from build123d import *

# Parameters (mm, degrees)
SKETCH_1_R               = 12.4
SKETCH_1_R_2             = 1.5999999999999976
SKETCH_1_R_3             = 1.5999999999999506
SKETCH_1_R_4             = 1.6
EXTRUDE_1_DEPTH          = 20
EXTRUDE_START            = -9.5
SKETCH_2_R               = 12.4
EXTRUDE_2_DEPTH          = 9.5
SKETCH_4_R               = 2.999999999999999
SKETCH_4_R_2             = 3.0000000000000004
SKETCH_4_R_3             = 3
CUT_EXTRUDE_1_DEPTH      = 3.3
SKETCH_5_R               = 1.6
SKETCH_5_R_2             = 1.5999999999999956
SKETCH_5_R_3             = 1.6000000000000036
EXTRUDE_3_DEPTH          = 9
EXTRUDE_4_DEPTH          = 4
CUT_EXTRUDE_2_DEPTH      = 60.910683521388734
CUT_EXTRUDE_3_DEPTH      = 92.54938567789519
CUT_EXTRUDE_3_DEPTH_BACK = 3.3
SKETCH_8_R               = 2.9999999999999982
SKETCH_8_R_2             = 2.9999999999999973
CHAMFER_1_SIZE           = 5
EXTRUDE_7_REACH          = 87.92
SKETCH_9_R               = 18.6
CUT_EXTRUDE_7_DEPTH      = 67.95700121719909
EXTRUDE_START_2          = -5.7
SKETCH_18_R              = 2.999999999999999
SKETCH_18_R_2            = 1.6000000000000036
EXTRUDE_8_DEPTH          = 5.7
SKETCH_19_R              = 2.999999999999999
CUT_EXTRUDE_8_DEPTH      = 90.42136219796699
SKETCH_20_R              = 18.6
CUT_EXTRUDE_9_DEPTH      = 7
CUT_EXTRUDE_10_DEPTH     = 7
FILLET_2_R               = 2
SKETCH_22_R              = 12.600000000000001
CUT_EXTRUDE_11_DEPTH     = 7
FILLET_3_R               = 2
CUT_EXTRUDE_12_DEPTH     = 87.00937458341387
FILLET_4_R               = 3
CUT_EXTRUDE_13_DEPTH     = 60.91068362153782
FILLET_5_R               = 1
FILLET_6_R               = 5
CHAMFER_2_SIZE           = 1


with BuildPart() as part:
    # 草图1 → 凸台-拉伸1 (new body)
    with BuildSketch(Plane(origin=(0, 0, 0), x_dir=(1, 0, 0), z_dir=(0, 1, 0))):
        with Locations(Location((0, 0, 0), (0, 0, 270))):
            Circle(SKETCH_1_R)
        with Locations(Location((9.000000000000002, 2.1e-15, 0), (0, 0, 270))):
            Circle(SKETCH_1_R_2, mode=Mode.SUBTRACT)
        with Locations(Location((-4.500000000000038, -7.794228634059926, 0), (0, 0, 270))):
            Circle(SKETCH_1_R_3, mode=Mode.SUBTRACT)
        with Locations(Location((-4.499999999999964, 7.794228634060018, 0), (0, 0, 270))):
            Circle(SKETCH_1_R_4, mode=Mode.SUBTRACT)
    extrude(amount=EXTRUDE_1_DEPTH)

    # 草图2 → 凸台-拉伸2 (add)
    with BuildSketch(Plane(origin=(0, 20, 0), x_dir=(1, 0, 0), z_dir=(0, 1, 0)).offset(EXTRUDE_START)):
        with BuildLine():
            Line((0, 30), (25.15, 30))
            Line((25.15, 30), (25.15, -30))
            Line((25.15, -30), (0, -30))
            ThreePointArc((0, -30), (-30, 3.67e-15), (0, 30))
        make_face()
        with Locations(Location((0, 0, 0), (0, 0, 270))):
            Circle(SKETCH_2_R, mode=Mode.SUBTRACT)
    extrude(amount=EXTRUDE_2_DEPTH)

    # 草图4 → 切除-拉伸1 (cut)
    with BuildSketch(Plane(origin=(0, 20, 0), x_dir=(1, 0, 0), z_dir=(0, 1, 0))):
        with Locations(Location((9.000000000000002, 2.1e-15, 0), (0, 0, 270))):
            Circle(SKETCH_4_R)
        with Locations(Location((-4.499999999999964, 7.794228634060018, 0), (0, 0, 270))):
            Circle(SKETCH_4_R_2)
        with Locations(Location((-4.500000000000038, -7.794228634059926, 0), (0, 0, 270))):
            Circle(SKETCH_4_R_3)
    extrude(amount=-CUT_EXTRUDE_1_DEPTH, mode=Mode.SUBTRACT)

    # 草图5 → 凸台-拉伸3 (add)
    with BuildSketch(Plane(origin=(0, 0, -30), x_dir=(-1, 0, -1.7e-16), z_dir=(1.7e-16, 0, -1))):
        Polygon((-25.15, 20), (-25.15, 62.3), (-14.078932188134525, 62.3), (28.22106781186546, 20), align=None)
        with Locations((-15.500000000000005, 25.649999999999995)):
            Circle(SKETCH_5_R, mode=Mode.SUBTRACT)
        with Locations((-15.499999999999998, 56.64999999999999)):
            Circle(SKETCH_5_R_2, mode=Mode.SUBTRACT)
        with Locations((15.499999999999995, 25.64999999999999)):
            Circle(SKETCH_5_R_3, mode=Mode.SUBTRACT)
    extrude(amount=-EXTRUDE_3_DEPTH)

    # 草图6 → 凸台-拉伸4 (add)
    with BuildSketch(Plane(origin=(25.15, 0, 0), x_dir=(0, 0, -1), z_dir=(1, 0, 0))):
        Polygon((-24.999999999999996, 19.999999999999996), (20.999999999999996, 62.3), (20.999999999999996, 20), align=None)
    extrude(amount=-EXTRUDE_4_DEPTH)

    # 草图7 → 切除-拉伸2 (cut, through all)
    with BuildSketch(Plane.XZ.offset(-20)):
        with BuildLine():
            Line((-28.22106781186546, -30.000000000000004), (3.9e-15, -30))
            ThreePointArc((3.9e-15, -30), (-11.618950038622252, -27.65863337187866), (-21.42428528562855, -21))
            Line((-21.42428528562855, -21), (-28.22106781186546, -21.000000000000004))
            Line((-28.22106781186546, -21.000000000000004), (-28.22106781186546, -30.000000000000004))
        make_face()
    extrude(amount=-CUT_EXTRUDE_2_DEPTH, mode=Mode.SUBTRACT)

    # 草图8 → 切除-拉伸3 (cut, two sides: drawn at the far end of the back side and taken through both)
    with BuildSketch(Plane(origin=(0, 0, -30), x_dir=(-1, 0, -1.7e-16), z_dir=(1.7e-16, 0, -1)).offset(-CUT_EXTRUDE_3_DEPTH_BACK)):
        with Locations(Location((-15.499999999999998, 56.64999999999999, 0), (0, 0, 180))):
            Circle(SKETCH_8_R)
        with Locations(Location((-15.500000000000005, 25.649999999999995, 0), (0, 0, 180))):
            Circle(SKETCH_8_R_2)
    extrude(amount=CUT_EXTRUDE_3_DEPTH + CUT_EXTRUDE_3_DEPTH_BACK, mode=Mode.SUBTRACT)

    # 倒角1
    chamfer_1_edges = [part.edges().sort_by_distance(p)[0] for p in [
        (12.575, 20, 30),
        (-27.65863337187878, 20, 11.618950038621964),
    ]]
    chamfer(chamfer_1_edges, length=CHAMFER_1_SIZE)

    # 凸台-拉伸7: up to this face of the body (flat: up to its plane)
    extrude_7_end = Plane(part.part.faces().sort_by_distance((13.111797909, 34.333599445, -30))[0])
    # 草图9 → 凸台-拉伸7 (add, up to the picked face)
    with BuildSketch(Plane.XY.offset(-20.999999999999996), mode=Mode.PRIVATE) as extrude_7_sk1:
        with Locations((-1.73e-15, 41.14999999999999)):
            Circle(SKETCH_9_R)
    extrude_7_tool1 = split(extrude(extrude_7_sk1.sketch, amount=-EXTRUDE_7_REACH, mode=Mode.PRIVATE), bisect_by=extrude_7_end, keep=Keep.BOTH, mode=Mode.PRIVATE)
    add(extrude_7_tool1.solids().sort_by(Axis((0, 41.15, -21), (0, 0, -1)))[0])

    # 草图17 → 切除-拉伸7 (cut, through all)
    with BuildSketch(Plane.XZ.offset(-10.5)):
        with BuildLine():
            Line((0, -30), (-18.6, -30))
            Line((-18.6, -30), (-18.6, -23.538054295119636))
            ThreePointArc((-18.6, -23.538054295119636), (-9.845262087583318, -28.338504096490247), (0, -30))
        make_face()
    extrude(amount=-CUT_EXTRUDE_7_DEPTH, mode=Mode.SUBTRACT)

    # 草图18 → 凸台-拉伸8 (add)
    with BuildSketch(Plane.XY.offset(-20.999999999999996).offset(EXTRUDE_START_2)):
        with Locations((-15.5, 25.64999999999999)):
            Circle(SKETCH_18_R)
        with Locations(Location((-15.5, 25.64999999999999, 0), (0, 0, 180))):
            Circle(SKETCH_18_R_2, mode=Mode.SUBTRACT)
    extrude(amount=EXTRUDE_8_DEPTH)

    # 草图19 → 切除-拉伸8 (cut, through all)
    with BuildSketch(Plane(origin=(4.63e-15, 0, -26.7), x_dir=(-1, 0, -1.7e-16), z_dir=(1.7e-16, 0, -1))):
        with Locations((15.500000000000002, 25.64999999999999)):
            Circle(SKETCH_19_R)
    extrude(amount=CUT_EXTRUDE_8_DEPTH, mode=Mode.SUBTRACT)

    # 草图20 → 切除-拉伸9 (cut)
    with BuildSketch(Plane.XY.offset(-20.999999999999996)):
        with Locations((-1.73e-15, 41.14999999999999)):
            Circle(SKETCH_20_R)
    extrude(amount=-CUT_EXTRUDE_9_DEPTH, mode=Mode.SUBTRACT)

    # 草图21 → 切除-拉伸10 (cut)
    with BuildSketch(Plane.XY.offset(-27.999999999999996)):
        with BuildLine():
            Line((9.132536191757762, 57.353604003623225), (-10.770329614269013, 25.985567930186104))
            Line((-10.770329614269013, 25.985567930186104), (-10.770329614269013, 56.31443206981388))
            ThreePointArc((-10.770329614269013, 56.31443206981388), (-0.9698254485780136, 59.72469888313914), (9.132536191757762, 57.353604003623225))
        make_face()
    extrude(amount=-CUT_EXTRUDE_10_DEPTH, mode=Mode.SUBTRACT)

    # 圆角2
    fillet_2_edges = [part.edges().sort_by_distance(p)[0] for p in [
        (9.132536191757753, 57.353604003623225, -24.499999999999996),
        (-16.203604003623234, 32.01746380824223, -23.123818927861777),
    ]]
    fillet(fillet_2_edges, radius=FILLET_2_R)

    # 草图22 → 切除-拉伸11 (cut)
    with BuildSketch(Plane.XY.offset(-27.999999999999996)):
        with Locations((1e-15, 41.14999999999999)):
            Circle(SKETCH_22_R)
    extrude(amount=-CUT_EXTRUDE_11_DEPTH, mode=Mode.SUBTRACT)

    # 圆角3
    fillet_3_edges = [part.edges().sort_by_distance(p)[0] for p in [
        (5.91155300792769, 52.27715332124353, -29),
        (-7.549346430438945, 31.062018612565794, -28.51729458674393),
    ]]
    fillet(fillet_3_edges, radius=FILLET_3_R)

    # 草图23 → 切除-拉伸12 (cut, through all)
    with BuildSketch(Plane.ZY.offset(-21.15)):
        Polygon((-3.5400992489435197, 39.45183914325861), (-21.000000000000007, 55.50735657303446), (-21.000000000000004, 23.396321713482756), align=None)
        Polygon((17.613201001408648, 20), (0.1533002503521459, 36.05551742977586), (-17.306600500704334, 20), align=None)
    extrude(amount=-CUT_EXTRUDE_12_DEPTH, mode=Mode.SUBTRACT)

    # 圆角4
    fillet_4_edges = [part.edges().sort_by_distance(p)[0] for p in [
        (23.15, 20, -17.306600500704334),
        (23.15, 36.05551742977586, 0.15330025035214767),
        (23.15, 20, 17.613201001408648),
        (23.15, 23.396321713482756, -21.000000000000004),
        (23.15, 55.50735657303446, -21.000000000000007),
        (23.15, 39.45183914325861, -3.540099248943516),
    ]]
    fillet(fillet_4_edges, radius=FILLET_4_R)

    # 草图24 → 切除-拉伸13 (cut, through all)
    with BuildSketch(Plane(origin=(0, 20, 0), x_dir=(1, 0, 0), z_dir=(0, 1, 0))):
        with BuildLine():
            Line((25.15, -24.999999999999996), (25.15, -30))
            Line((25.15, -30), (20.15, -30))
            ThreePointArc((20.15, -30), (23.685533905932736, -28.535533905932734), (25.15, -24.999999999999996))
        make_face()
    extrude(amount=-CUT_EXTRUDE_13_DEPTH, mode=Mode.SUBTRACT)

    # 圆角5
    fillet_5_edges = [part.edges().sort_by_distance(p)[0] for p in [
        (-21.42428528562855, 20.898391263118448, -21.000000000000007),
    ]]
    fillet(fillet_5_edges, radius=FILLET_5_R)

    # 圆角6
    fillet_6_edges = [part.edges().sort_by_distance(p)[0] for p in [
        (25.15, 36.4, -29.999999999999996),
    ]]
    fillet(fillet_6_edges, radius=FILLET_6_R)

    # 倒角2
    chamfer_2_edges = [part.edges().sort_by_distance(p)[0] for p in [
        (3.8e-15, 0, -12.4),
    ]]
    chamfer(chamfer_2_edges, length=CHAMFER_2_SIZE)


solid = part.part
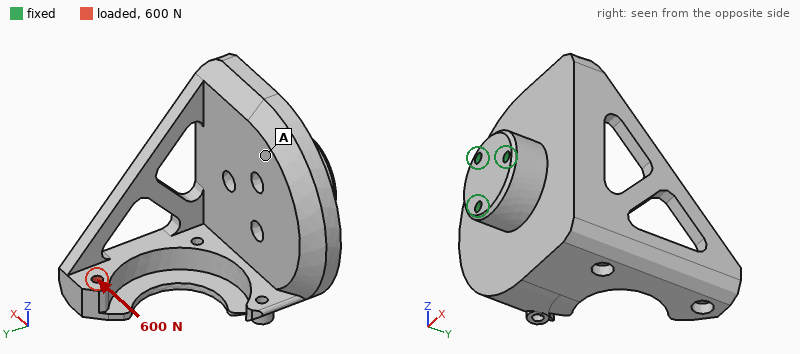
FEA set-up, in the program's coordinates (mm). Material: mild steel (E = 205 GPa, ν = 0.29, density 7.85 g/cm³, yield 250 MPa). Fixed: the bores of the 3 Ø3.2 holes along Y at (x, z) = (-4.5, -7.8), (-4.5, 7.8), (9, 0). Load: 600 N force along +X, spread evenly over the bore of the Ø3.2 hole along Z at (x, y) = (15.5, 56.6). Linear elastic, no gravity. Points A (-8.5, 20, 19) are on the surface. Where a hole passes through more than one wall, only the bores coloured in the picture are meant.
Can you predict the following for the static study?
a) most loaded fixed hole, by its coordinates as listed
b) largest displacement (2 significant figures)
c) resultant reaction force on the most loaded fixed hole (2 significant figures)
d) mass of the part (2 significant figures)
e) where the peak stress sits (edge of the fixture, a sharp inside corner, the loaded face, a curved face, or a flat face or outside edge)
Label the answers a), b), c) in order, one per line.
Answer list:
a) (9, 0)
b) 91 µm
c) 1.3 kN
d) 300 g
e) a curved face
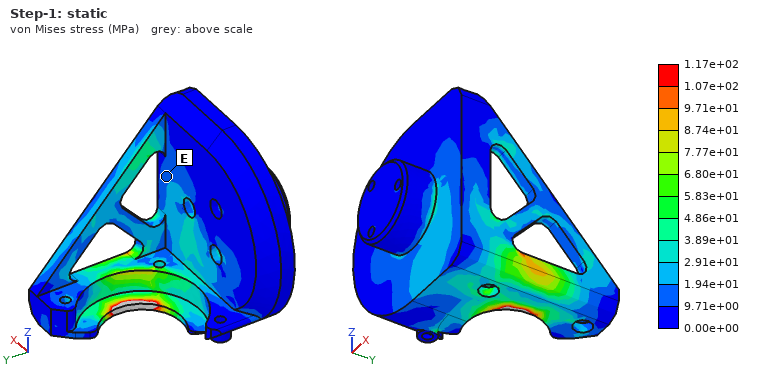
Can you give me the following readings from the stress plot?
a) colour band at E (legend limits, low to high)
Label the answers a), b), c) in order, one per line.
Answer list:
a) 9.71e+00 to 1.94e+01 MPa
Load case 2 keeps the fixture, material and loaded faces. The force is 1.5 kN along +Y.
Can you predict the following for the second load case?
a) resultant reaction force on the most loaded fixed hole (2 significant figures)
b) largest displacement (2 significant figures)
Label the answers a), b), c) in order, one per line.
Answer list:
a) 1.2 kN
b) 40 µm
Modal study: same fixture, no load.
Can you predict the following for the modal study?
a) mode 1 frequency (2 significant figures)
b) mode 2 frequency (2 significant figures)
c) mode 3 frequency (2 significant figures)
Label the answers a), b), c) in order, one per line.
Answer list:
a) 3400 Hz
b) 4700 Hz
c) 6900 Hz
